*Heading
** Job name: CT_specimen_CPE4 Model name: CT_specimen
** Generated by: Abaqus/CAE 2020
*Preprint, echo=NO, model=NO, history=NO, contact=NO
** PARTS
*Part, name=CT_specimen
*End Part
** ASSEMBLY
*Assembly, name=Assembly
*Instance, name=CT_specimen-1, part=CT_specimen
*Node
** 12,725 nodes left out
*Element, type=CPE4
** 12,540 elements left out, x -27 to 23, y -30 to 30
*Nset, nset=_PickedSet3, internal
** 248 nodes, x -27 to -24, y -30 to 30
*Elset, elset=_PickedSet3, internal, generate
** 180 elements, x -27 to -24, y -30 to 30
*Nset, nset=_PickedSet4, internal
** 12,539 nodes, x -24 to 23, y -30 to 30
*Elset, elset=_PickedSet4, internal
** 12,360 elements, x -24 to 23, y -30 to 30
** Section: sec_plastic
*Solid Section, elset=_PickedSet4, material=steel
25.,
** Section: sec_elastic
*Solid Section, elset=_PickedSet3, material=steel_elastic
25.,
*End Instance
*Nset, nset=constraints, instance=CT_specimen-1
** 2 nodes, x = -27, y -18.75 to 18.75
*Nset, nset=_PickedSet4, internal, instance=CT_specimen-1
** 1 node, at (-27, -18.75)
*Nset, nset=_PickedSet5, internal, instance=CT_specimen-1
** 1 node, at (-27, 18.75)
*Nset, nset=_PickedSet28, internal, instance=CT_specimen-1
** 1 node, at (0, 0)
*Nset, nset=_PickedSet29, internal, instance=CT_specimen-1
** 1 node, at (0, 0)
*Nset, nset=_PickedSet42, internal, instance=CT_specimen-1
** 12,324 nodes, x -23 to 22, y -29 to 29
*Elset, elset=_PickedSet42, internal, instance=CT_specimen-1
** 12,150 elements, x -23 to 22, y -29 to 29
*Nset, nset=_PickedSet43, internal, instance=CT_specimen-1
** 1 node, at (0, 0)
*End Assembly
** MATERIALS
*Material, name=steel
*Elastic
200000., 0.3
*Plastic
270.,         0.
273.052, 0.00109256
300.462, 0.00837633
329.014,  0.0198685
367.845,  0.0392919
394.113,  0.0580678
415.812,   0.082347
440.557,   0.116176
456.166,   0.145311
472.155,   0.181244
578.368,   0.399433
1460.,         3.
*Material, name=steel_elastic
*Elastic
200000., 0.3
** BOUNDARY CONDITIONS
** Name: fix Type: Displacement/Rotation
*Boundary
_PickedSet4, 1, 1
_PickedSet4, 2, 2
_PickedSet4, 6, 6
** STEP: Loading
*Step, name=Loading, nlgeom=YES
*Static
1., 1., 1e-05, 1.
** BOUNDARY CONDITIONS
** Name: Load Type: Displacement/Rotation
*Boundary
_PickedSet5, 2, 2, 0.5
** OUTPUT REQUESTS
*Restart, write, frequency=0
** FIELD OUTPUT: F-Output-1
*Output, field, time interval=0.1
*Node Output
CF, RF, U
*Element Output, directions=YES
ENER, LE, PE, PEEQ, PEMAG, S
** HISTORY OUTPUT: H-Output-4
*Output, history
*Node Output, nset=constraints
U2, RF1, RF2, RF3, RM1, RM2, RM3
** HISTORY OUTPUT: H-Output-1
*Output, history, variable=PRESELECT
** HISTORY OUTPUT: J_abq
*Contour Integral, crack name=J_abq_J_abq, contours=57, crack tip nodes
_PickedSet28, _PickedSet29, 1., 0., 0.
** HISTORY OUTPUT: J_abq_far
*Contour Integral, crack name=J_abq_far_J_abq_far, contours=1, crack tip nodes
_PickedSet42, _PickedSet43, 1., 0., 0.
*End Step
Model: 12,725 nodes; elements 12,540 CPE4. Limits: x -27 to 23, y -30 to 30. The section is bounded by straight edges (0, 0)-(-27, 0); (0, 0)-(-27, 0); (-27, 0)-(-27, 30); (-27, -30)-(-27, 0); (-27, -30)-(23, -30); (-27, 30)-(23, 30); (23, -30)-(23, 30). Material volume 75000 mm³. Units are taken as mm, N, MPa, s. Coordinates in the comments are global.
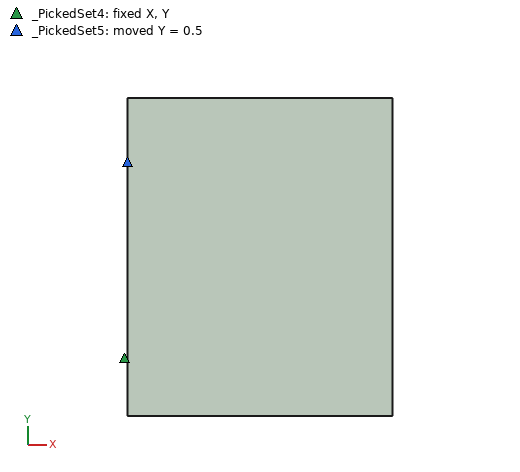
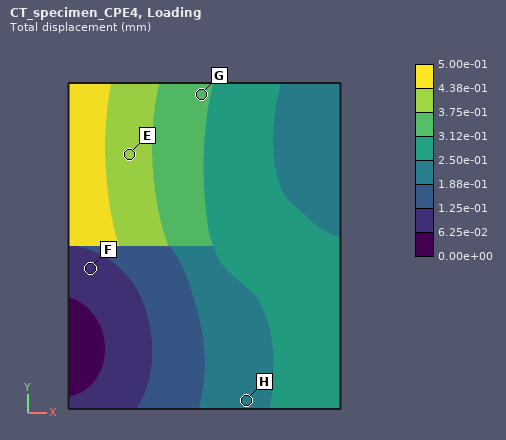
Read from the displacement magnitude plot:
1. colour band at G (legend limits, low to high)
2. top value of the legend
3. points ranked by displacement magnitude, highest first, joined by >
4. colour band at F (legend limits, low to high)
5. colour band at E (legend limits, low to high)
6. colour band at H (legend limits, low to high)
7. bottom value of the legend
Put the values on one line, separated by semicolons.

3.12e-01 to 3.75e-01 mm; 5.00e-01 mm; E > G > H > F; 6.25e-02 to 1.25e-01 mm; 3.75e-01 to 4.38e-01 mm; 1.88e-01 to 2.50e-01 mm; 0.00e+00 mm
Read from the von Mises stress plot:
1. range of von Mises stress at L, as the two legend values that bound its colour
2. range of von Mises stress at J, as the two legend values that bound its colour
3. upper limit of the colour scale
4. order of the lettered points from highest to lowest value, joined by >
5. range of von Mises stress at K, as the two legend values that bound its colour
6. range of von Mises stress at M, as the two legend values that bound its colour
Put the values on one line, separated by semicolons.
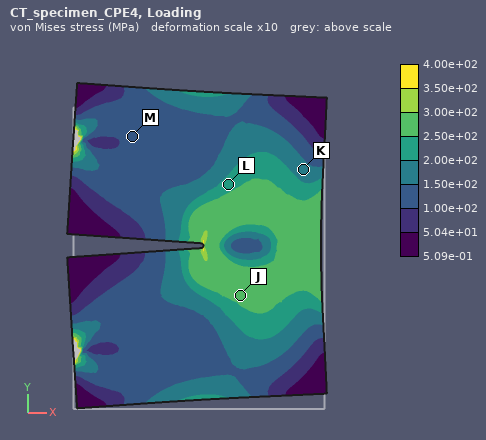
2.00e+02 to 2.50e+02 MPa; 2.50e+02 to 3.00e+02 MPa; 4.00e+02 MPa; J > L > K > M; 1.50e+02 to 2.00e+02 MPa; 1.00e+02 to 1.50e+02 MPa
